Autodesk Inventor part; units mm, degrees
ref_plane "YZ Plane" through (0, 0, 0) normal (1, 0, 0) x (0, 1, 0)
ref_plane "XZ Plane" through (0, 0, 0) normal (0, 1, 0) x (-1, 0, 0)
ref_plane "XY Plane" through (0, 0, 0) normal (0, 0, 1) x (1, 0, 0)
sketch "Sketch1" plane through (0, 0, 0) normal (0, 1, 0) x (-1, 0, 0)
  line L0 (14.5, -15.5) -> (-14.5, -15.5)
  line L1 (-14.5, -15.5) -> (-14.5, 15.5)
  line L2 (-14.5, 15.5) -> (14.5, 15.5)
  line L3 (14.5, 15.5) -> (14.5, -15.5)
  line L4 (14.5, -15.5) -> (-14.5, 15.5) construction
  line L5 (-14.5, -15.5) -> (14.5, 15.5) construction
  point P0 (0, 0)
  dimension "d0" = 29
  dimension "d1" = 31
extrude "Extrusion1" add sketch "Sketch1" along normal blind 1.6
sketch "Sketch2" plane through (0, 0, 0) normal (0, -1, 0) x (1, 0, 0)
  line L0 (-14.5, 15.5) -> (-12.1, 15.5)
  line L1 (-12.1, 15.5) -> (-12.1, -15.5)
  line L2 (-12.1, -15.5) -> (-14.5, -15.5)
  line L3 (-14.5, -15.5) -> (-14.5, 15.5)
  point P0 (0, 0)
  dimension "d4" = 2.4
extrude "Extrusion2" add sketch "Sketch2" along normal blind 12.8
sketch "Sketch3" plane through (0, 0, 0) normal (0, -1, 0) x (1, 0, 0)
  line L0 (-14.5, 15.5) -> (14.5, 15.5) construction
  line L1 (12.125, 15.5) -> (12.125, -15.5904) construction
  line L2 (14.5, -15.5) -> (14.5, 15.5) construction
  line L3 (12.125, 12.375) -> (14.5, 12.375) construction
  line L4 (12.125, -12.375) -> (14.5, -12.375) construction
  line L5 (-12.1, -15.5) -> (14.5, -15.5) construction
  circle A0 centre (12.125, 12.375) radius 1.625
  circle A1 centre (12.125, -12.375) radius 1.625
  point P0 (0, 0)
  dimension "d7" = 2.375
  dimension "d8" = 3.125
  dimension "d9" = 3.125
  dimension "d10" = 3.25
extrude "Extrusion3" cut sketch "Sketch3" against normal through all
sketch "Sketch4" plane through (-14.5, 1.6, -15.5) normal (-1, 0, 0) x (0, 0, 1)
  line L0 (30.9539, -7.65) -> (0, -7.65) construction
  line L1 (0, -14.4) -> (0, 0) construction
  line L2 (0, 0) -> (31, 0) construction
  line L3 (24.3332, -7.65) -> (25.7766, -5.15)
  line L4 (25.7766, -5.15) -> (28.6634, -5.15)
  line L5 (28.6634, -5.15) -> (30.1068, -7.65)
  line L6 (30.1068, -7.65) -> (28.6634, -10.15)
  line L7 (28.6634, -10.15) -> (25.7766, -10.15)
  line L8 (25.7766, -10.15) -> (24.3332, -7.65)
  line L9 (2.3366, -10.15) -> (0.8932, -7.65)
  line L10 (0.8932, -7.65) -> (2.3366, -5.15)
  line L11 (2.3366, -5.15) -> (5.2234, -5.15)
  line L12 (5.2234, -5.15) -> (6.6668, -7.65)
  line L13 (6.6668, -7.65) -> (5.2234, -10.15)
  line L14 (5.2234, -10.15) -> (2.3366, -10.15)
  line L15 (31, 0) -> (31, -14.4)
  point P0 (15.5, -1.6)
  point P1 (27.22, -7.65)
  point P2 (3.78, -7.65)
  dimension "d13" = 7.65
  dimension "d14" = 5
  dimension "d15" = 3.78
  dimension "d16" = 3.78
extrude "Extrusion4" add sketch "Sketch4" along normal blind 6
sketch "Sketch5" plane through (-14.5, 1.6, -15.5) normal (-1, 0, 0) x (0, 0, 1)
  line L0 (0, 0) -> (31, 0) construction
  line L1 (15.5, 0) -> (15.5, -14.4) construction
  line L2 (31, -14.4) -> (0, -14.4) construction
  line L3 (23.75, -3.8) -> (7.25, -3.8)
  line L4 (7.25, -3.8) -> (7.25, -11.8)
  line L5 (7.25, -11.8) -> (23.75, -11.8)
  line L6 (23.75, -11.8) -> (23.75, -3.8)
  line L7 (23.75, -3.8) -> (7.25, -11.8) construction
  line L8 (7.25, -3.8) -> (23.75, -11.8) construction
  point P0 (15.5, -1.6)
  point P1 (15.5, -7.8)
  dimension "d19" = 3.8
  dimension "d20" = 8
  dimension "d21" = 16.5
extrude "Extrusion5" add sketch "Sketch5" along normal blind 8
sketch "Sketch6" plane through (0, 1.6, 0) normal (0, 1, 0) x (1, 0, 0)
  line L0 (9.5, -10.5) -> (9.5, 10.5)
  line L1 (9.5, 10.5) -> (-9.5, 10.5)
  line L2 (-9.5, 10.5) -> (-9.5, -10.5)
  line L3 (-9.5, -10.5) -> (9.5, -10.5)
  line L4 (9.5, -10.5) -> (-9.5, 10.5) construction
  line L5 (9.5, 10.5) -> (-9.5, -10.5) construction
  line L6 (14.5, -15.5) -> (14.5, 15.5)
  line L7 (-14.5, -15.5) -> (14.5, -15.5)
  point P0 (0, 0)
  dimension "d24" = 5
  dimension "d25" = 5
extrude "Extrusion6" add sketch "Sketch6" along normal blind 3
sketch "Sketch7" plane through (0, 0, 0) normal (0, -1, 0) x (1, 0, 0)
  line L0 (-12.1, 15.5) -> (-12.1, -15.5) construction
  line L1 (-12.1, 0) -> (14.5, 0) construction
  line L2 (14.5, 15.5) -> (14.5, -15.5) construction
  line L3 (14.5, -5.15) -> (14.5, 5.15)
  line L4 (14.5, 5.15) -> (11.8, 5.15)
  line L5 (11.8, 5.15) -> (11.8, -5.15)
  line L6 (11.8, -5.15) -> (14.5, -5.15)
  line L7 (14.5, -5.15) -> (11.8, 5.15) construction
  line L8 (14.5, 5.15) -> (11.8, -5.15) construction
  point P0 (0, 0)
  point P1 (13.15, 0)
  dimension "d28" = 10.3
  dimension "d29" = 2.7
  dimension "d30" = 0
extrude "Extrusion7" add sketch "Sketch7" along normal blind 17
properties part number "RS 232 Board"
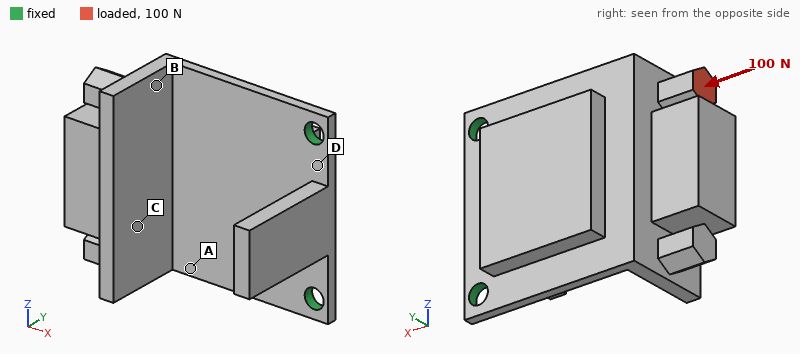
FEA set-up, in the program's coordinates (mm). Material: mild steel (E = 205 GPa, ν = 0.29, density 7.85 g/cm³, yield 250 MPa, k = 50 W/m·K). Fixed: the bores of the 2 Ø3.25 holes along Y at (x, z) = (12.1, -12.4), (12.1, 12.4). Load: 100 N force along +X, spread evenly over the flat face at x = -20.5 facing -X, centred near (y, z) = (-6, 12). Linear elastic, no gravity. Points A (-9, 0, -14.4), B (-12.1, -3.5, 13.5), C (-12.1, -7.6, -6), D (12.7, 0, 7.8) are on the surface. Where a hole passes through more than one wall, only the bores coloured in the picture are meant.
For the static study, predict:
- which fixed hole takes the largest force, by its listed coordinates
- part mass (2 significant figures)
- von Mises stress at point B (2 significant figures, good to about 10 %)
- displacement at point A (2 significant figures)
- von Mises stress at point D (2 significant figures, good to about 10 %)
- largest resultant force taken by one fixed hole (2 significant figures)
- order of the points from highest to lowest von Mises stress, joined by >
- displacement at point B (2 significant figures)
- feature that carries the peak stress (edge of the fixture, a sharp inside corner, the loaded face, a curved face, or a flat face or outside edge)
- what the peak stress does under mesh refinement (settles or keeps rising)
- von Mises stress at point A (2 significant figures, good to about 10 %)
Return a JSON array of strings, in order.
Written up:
["(12.1, 12.4)", "42 g", "13 MPa", "29 µm", "35 MPa", "100 N", "D > A > B > C", "41 µm", "edge of the fixture", "keeps rising", "24 MPa"]
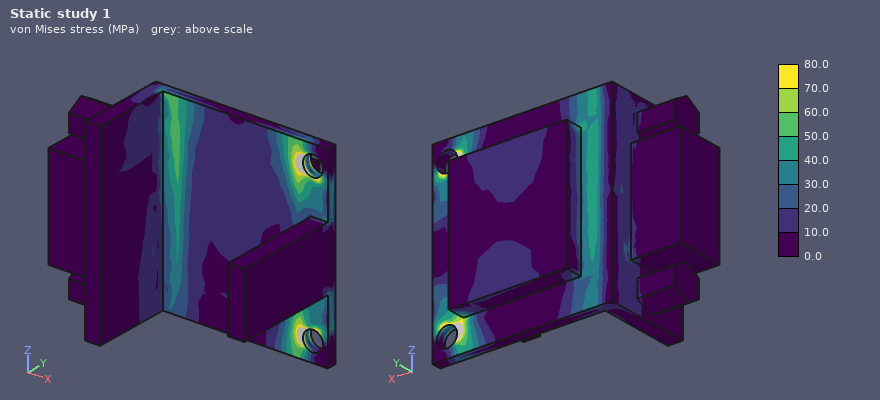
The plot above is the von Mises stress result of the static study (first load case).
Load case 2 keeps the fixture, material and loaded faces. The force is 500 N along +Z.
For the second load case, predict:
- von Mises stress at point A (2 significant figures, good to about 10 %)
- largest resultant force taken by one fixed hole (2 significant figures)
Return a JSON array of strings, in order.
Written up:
["31 MPa", "700 N"]
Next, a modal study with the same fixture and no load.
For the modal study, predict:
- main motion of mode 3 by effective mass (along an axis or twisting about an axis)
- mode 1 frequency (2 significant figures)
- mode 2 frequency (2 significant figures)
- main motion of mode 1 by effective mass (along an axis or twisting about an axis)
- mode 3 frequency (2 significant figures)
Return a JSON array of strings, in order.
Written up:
["along Z", "800 Hz", "3500 Hz", "along Y", "3700 Hz"]
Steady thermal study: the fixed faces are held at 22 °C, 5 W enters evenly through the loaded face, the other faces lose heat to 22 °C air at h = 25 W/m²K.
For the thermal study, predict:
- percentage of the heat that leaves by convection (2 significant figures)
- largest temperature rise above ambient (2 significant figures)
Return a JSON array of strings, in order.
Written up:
["40 %", "73 K"]
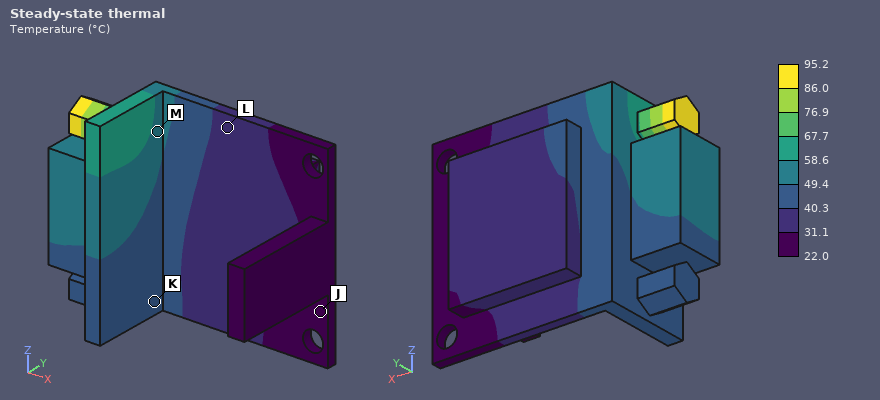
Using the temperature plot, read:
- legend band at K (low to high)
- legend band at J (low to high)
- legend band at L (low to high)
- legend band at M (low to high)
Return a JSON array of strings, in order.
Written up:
["40.3 to 49.4 °C", "22.0 to 31.1 °C", "31.1 to 40.3 °C", "49.4 to 58.6 °C"]
